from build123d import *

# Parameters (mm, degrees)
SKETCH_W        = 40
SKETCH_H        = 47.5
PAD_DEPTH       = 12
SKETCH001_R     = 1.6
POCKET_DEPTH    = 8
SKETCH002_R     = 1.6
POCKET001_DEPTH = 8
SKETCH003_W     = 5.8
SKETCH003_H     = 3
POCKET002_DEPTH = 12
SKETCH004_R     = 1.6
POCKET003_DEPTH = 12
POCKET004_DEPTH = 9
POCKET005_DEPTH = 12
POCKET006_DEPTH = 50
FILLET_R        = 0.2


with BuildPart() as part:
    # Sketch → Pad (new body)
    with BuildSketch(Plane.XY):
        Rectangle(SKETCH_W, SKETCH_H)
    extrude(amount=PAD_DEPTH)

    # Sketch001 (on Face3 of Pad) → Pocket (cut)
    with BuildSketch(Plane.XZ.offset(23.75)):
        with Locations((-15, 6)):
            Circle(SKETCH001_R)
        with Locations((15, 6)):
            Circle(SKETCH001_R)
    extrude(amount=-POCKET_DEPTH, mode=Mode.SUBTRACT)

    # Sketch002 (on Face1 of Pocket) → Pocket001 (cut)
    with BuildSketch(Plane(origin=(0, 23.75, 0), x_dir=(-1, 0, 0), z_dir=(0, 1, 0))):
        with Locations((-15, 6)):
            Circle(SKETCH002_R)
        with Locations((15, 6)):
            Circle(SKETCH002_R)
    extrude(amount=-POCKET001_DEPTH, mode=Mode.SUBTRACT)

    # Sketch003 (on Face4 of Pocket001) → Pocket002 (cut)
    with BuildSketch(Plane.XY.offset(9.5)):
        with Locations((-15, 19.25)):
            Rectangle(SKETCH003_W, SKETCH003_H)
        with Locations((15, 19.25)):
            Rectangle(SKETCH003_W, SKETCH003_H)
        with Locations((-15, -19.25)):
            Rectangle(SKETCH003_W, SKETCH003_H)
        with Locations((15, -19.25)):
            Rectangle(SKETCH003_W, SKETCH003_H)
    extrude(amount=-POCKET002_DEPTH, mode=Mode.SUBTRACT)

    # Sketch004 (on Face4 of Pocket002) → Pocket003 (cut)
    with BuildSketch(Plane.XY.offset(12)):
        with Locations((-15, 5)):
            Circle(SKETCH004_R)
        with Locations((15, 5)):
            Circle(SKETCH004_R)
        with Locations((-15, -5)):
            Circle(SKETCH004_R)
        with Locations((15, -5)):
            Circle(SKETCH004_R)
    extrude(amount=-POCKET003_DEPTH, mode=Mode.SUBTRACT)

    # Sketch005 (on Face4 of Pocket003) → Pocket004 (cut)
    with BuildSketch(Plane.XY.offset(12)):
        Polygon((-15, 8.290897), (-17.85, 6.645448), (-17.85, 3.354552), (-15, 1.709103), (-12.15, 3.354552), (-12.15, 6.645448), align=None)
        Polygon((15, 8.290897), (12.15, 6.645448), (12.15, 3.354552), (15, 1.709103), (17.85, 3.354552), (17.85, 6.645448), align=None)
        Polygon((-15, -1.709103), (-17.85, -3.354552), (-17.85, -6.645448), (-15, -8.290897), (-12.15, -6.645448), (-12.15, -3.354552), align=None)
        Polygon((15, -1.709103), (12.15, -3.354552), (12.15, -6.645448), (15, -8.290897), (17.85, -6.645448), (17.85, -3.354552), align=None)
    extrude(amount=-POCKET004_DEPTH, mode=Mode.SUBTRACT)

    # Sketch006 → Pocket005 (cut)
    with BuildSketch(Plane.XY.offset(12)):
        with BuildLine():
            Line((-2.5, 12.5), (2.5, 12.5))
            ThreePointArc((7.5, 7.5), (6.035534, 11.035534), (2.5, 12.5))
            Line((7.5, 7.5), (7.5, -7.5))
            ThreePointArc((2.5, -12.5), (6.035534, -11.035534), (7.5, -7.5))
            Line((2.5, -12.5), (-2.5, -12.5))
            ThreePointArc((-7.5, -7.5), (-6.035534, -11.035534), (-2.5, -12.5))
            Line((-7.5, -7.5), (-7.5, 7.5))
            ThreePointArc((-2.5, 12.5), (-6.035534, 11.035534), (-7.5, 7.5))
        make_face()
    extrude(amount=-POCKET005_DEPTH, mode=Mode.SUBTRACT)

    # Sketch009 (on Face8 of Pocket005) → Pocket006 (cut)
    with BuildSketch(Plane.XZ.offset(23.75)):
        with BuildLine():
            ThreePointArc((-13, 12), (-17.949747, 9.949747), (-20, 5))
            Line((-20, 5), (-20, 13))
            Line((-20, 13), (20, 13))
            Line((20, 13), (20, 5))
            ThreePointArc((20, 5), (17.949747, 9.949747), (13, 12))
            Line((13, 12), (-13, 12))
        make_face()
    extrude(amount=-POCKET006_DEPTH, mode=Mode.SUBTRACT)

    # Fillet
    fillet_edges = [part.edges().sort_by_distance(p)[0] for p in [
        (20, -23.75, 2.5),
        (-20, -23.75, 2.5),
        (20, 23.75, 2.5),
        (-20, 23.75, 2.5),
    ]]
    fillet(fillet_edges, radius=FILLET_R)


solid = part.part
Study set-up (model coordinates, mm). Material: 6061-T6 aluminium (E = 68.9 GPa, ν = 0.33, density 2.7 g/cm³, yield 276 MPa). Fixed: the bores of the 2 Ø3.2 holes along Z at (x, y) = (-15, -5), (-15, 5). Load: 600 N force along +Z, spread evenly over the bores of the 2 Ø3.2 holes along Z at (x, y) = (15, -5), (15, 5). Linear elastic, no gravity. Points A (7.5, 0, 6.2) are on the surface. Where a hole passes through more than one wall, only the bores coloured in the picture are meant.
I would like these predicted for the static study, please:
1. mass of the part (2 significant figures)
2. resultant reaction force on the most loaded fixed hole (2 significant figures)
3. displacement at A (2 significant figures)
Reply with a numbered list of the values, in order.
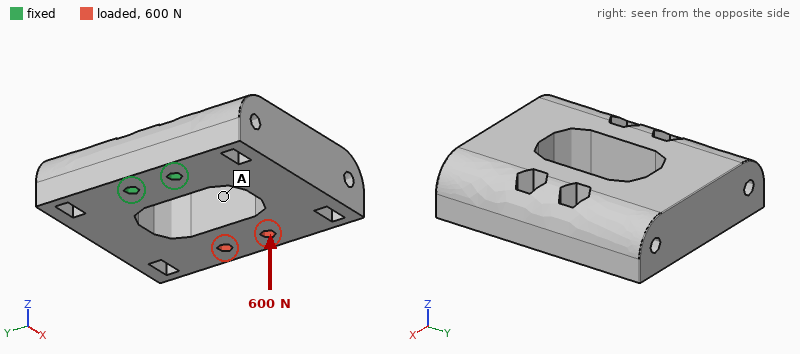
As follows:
1. 42 g
2. 310 N
3. 0.14 mm
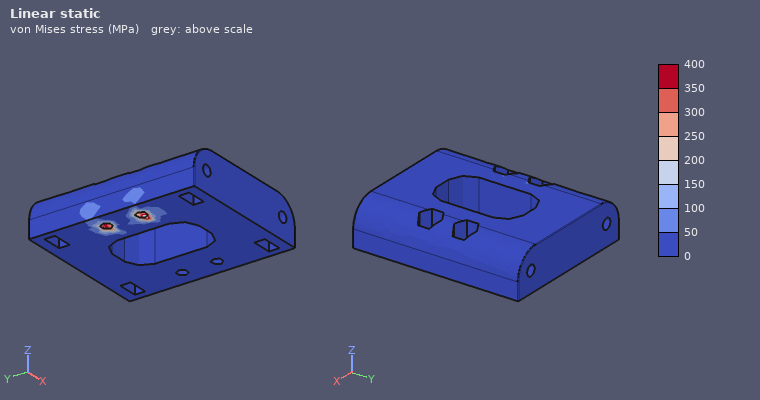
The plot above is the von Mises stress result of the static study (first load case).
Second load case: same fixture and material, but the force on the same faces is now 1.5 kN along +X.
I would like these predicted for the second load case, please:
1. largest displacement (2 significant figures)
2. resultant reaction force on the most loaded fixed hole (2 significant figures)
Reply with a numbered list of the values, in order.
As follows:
1. 38 µm
2. 760 N
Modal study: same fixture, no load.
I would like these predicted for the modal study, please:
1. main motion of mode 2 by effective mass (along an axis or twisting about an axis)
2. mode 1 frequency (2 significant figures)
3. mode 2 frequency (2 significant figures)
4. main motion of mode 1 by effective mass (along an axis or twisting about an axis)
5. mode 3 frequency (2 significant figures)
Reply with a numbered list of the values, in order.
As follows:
1. along Y
2. 2100 Hz
3. 3700 Hz
4. along Z
5. 4600 Hz
